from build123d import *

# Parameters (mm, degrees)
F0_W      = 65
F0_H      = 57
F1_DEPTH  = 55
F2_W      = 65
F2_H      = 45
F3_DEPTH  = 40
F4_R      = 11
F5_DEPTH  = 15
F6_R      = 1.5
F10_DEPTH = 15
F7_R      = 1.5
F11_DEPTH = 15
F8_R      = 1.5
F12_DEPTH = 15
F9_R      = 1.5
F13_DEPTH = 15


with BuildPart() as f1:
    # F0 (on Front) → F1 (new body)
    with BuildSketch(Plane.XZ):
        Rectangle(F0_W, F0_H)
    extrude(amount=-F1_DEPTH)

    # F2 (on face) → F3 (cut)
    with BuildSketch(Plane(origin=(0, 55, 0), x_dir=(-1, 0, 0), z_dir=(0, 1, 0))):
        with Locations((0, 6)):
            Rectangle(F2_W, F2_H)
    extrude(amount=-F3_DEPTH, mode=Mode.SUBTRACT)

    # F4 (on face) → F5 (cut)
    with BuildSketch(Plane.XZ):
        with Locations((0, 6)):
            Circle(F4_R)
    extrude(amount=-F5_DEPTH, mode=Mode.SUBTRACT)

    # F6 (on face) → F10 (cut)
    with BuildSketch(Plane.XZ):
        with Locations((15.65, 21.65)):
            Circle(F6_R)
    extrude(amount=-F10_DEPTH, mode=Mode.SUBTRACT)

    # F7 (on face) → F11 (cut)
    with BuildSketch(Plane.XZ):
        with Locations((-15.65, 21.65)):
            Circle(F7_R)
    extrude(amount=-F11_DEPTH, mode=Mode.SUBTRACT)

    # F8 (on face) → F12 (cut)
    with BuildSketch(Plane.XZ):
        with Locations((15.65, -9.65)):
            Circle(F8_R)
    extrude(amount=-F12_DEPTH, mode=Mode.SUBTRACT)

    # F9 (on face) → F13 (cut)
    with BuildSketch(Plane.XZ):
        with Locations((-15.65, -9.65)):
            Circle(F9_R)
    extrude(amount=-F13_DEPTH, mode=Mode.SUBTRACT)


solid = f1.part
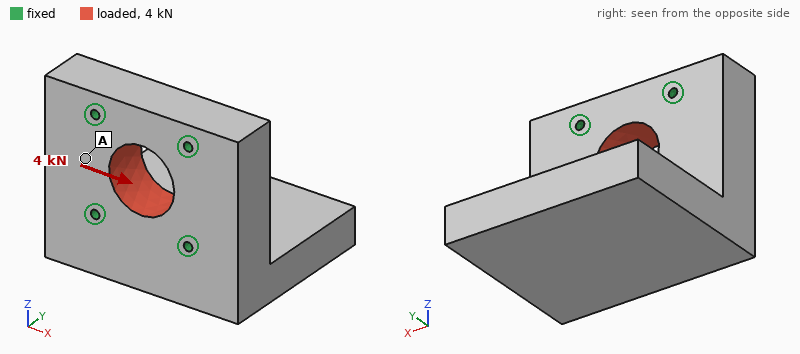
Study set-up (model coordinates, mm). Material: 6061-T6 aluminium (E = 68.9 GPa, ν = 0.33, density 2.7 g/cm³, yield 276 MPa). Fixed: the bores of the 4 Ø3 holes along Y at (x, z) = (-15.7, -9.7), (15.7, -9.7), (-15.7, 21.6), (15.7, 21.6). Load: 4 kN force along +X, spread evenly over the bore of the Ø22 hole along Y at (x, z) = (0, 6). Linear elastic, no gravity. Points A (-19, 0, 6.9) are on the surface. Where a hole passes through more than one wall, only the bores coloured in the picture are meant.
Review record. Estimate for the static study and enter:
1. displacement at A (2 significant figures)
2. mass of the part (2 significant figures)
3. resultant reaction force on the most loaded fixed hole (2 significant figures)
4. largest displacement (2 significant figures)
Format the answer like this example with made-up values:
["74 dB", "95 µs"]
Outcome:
["1.2 µm", "220 g", "1.0 kN", "1.6 µm"]
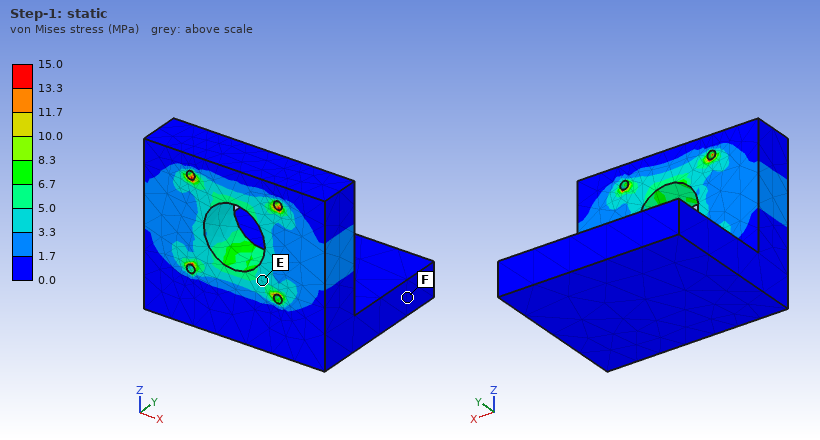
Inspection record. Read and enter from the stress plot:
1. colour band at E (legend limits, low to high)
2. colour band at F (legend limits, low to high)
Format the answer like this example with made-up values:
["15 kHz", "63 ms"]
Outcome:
["3.3 to 5.0 MPa", "0.0 to 1.7 MPa"]
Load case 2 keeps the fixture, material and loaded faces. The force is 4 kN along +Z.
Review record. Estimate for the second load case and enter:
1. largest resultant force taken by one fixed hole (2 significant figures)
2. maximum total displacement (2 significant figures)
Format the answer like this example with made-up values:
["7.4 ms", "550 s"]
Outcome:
["1.0 kN", "2.3 µm"]
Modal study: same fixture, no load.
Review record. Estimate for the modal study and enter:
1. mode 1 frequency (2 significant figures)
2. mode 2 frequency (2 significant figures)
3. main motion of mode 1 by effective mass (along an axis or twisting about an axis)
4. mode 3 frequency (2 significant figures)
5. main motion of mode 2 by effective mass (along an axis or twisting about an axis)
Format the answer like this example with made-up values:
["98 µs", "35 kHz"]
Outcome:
["3400 Hz", "6100 Hz", "along Z", "7800 Hz", "along X"]
